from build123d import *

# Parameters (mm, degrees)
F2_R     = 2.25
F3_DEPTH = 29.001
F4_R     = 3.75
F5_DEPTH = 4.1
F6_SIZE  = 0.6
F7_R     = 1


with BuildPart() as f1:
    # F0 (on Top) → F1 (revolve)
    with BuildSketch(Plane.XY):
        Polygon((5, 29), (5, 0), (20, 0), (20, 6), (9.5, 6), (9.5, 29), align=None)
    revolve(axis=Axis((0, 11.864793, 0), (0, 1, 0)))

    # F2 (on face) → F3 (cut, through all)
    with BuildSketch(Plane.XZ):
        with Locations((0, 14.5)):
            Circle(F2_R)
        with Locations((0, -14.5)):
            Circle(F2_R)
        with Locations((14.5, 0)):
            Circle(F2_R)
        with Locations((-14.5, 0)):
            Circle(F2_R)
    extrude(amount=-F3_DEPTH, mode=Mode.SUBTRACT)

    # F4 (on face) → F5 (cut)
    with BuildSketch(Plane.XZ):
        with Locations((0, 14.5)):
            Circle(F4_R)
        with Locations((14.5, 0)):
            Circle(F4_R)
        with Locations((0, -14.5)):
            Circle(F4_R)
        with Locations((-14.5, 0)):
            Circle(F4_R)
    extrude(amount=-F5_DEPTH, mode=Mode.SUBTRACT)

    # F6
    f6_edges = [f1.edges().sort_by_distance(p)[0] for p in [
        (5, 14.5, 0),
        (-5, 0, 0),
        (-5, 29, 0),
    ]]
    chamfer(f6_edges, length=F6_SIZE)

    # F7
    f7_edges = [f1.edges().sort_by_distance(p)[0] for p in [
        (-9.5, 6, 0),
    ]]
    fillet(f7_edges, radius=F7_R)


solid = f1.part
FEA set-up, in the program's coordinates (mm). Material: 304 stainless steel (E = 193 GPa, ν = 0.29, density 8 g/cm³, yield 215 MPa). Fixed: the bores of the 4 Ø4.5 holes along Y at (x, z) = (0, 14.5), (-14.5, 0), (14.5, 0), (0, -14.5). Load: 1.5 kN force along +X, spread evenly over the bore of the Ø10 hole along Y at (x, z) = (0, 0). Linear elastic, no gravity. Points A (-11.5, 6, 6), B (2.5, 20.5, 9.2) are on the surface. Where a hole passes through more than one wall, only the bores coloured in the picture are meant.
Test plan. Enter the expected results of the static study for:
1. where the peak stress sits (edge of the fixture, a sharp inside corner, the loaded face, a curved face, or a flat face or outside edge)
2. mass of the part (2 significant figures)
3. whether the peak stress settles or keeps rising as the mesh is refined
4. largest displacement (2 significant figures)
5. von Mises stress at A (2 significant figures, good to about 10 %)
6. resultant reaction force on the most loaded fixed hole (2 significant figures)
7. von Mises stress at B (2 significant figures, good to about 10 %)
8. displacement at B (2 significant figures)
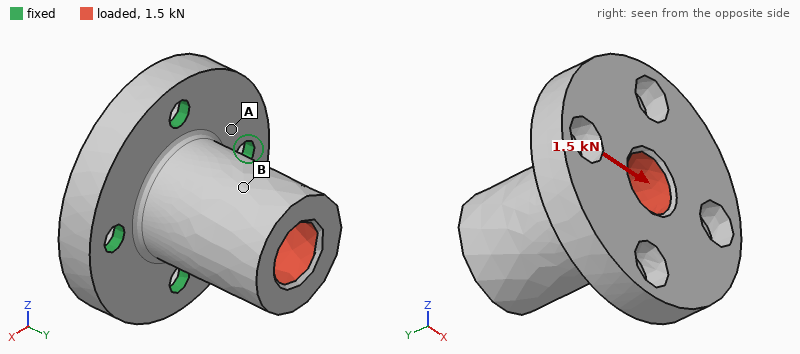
edge of the fixture
88 g
keeps rising
7.6 µm
12 MPa
620 N
5.5 MPa
4.8 µm
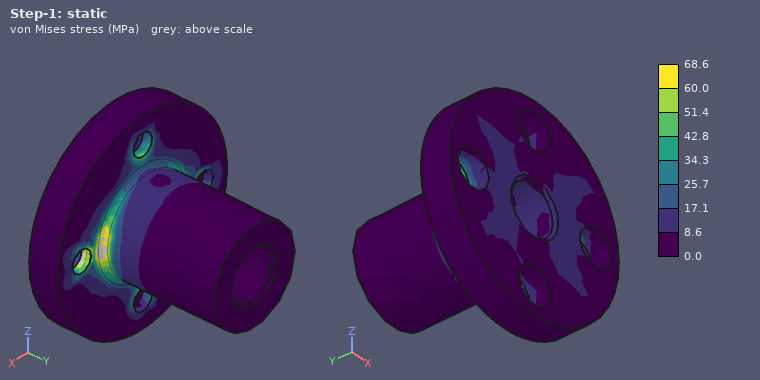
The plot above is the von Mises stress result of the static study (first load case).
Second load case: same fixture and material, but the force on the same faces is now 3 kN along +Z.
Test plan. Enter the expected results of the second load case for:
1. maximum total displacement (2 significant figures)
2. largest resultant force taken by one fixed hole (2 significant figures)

15 µm
1.2 kN
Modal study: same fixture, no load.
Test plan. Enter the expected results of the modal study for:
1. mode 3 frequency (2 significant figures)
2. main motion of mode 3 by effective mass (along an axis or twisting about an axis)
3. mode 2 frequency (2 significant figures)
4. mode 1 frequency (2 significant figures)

21 kHz
along Y
12 kHz
12 kHz
